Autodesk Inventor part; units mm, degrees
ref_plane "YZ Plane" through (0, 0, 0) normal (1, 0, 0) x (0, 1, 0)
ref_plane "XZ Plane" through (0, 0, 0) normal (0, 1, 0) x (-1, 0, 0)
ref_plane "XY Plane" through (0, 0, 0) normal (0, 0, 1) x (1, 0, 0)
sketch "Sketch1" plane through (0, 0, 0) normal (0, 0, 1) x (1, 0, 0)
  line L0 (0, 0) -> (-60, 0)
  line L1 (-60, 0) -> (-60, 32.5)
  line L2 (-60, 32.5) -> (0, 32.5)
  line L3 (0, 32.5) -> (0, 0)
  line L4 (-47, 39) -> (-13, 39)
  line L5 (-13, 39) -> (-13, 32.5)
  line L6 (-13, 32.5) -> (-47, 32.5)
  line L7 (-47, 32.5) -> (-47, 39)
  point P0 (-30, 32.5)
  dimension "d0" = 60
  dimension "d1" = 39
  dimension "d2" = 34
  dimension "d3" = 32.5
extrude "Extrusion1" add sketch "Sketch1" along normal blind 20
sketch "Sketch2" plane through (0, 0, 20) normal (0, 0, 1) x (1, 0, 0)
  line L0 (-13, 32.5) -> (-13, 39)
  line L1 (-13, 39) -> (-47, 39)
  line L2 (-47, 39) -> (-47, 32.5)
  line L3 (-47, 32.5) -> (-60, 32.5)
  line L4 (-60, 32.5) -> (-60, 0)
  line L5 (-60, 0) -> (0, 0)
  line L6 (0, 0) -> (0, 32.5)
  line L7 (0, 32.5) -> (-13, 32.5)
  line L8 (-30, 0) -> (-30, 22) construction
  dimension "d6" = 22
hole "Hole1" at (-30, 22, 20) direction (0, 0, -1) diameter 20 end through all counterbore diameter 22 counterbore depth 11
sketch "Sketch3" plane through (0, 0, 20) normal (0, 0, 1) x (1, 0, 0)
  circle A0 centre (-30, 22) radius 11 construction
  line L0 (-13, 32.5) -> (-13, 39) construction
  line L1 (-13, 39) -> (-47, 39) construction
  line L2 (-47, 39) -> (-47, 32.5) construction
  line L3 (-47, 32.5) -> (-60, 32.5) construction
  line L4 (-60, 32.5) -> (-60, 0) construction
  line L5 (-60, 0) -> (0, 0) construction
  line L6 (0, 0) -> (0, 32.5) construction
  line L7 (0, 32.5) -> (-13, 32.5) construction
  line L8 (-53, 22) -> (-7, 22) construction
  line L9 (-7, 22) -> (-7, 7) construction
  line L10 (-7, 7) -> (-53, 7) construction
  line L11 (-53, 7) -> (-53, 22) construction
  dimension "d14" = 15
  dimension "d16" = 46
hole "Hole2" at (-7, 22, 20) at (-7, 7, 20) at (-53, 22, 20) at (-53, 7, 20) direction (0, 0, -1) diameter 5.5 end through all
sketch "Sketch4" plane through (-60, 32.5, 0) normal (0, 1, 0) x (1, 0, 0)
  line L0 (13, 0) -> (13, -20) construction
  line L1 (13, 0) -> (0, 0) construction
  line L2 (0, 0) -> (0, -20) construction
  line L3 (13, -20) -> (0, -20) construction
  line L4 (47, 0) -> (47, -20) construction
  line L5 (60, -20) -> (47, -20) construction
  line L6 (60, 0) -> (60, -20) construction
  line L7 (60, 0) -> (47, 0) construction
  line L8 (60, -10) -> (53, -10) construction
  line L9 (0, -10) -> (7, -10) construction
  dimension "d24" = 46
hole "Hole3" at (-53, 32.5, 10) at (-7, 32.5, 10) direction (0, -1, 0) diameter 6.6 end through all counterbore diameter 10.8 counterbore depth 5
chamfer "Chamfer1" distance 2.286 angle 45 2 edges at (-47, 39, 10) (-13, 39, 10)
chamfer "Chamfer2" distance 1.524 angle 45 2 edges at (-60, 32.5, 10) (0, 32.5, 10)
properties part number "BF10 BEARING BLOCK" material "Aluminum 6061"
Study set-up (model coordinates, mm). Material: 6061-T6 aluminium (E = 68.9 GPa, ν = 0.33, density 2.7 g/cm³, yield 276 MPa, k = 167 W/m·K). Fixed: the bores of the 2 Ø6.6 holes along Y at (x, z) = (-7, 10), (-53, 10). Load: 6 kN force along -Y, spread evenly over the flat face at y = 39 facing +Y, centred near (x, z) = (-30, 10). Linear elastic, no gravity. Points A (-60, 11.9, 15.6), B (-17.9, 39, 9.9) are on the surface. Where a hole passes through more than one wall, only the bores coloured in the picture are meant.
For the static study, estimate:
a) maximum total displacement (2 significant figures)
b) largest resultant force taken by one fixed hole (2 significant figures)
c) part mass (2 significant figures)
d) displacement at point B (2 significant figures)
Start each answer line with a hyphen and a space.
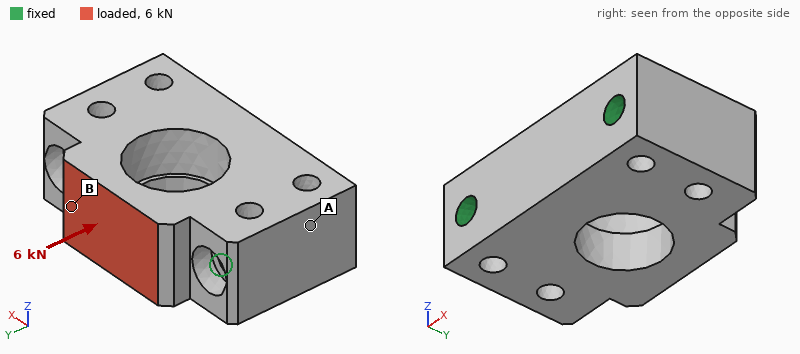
- 13 µm
- 3.4 kN
- 87 g
- 6.4 µm
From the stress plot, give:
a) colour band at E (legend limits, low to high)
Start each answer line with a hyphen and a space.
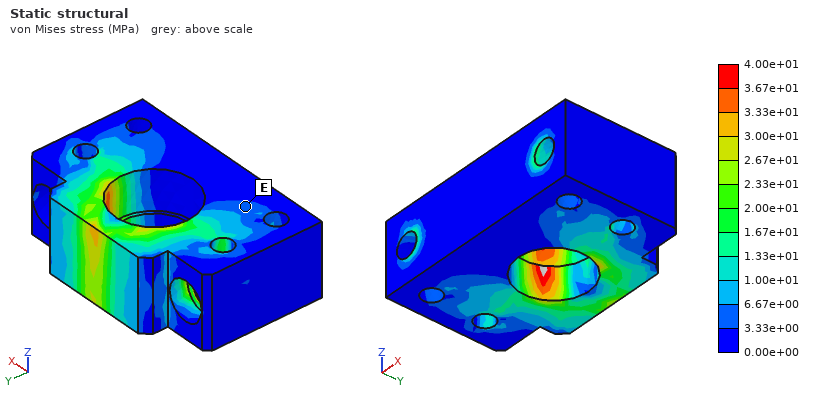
- 3.33e+00 to 6.67e+00 MPa
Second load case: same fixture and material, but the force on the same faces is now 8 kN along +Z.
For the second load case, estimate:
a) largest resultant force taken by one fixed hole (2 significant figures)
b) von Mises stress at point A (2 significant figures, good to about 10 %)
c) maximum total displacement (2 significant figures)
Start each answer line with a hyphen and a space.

- 4.0 kN
- 16 MPa
- 74 µm
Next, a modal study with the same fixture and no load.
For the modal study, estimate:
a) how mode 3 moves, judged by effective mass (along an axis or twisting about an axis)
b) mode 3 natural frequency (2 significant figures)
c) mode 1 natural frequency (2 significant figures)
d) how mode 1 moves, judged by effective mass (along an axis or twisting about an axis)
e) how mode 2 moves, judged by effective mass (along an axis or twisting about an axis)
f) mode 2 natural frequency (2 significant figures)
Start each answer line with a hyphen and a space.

- along X
- 29 kHz
- 17 kHz
- along Z
- along Z
- 25 kHz
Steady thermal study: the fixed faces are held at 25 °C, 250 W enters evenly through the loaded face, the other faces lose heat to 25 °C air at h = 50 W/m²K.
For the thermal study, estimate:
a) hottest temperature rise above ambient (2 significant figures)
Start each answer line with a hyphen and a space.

- 77 K
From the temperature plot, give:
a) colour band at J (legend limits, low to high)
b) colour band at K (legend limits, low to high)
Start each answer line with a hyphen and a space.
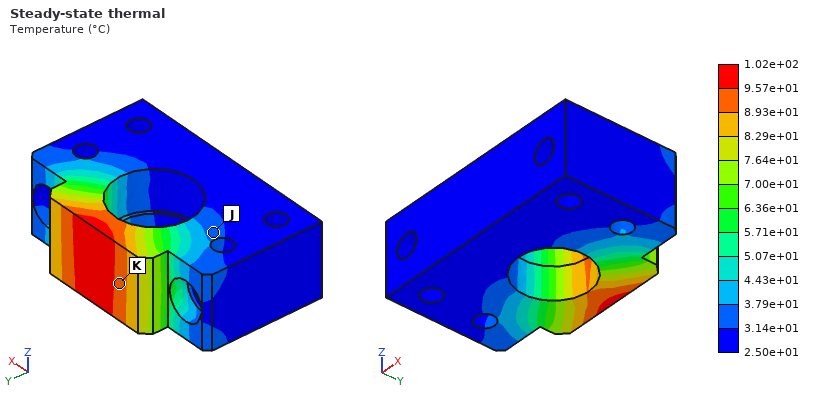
- 3.14e+01 to 3.79e+01 °C
- 8.93e+01 to 9.57e+01 °C
